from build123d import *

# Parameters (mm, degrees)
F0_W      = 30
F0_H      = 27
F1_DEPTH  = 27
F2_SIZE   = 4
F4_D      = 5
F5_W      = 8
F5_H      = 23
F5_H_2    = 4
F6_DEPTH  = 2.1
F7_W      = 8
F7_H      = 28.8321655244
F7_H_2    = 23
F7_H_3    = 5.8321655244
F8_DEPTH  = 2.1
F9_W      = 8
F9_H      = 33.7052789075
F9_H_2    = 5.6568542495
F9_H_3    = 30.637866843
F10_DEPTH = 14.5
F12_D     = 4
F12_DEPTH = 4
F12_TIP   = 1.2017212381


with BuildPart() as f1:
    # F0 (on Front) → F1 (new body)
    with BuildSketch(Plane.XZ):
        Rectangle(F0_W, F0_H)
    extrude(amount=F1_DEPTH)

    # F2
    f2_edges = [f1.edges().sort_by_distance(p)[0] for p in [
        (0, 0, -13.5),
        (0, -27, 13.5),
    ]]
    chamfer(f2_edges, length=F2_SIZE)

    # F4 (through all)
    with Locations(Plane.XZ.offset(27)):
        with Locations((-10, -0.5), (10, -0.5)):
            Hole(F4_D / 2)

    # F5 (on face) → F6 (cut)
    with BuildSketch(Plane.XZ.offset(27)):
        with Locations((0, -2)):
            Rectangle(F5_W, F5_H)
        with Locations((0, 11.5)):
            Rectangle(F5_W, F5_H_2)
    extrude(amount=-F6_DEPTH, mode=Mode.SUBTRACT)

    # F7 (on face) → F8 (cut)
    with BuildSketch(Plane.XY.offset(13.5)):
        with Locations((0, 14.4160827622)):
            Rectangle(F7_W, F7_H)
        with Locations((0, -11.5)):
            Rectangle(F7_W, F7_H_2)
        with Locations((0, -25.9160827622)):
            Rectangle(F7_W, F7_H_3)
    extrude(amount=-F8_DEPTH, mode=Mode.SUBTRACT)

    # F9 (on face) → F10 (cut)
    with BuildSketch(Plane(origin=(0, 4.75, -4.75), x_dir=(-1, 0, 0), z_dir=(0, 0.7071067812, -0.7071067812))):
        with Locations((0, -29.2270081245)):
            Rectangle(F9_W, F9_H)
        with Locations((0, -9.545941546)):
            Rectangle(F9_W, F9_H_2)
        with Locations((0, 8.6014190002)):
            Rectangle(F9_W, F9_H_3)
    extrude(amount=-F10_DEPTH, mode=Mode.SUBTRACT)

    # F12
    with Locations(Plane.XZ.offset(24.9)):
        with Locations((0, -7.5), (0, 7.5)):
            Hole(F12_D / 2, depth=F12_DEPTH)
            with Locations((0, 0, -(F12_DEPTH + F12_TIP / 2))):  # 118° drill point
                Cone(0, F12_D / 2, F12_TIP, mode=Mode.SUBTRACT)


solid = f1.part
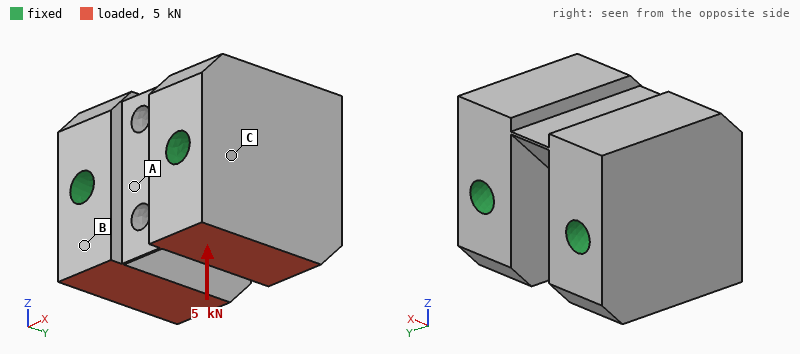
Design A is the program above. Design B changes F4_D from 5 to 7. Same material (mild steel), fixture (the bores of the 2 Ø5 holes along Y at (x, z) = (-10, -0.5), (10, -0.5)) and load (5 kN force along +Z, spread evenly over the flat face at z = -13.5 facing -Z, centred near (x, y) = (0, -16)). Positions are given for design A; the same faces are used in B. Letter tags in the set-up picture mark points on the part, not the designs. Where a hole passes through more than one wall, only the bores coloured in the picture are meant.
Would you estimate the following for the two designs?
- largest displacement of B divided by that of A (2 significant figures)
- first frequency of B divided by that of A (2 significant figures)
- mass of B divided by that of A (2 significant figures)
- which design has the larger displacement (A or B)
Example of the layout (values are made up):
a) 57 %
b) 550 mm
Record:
a) 0.89
b) 1.2
c) 0.94
d) A
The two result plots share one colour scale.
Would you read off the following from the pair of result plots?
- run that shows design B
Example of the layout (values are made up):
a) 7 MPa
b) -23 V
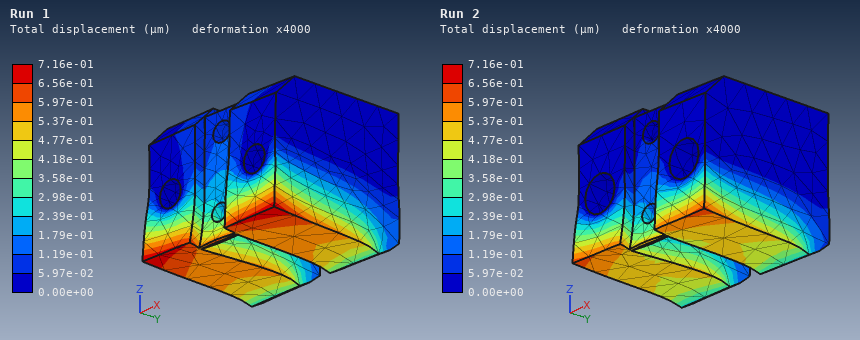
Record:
a) Run 2
